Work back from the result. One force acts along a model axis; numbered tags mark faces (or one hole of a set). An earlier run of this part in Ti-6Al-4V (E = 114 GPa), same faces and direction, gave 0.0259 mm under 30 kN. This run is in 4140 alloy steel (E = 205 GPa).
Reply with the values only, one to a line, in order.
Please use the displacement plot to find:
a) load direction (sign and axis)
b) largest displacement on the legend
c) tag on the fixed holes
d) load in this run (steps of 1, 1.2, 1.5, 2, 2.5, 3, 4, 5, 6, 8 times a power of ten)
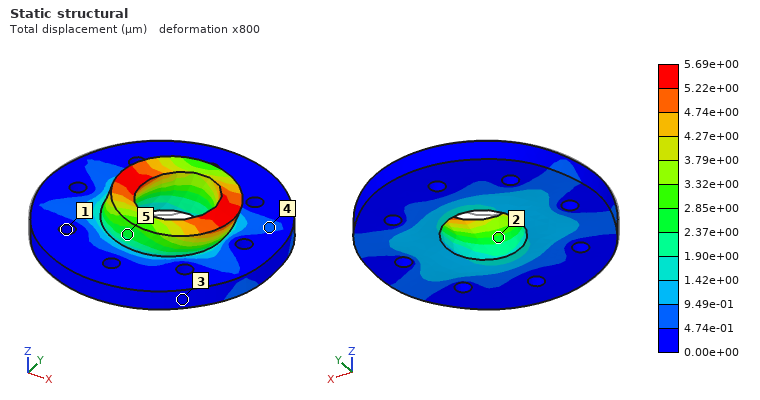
+X
5.69e+00 µm
1
12 kN
